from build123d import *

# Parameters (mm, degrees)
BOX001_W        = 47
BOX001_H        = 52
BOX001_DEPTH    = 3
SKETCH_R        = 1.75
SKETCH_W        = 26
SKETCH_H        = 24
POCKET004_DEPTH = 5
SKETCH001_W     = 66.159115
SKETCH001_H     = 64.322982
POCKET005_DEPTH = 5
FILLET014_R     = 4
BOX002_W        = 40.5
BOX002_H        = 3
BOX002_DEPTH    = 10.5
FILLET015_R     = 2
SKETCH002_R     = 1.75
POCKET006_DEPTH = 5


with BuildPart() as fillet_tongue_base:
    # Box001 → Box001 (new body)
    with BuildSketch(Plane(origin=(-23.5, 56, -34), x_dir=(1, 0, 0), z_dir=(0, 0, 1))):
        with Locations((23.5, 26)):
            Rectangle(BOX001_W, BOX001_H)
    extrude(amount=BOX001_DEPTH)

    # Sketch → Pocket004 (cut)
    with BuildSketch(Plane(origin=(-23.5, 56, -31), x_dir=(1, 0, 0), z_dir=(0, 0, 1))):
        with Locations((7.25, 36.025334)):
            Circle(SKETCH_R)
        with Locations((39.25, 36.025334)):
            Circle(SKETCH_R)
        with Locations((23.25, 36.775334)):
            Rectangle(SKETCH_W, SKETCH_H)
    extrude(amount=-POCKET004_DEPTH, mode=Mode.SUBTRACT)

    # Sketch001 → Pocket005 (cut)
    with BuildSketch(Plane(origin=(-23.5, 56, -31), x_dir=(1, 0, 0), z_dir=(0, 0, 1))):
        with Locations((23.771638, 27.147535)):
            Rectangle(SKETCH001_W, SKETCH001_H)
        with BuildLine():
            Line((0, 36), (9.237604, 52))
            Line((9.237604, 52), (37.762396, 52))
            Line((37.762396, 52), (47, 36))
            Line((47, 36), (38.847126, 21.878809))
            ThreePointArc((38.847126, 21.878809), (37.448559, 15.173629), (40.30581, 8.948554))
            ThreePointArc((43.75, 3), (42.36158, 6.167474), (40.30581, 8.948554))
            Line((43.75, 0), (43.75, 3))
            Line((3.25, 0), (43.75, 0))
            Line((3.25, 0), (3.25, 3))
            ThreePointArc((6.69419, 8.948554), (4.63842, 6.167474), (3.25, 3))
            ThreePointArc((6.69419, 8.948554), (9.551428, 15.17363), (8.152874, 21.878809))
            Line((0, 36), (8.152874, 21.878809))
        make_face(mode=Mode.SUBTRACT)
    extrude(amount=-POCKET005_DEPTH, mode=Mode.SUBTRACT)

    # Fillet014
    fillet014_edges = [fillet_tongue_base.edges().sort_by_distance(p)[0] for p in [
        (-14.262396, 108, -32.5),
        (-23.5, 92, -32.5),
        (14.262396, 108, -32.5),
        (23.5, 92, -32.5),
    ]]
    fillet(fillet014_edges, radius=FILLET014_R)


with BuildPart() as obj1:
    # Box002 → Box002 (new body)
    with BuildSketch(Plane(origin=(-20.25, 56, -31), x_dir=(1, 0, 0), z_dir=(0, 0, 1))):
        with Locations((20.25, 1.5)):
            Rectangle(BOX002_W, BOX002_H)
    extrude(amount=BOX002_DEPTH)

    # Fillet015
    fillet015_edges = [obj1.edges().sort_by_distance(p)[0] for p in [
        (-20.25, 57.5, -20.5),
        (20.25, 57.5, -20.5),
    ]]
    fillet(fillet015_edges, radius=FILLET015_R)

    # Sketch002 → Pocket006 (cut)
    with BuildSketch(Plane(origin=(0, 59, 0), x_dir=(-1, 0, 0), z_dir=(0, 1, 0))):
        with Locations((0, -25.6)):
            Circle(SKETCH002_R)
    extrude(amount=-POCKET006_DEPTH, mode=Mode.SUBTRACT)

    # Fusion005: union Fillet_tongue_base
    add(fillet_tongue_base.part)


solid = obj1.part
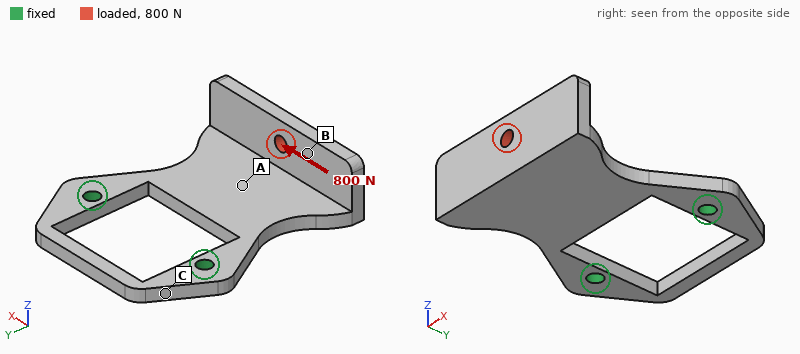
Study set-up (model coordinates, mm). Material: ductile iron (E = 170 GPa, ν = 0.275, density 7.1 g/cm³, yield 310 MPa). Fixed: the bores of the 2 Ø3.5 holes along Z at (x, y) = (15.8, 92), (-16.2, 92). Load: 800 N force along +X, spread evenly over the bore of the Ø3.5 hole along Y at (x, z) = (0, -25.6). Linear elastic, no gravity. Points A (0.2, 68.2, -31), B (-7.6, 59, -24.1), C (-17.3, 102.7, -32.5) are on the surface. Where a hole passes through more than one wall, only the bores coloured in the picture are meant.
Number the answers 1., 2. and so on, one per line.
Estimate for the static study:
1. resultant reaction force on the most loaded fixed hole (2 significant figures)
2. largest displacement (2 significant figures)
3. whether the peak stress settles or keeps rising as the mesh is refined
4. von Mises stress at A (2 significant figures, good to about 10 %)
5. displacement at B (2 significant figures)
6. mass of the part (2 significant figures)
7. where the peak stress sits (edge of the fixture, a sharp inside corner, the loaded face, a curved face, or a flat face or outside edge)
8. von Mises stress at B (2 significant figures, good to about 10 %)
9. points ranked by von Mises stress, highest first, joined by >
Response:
1. 790 N
2. 0.19 mm
3. keeps rising
4. 110 MPa
5. 0.11 mm
6. 35 g
7. edge of the fixture
8. 39 MPa
9. A > B > C
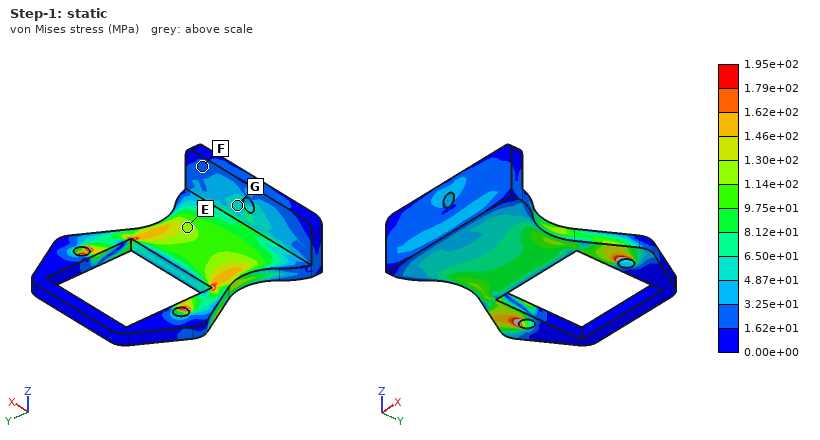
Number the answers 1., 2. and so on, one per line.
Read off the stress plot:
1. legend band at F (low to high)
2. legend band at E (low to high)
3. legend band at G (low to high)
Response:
1. 1.62e+01 to 3.25e+01 MPa
2. 1.14e+02 to 1.30e+02 MPa
3. 4.87e+01 to 6.50e+01 MPa
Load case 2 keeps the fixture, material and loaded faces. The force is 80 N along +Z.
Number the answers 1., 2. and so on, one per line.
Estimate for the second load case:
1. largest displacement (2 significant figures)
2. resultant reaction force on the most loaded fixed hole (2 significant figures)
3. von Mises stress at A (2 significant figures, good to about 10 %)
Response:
1. 0.26 mm
2. 40 N
3. 19 MPa
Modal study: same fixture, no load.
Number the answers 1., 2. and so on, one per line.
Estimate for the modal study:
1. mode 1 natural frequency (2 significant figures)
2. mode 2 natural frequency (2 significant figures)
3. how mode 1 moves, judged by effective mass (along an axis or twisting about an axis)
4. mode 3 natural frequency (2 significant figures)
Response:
1. 730 Hz
2. 2500 Hz
3. along Z
4. 5400 Hz
